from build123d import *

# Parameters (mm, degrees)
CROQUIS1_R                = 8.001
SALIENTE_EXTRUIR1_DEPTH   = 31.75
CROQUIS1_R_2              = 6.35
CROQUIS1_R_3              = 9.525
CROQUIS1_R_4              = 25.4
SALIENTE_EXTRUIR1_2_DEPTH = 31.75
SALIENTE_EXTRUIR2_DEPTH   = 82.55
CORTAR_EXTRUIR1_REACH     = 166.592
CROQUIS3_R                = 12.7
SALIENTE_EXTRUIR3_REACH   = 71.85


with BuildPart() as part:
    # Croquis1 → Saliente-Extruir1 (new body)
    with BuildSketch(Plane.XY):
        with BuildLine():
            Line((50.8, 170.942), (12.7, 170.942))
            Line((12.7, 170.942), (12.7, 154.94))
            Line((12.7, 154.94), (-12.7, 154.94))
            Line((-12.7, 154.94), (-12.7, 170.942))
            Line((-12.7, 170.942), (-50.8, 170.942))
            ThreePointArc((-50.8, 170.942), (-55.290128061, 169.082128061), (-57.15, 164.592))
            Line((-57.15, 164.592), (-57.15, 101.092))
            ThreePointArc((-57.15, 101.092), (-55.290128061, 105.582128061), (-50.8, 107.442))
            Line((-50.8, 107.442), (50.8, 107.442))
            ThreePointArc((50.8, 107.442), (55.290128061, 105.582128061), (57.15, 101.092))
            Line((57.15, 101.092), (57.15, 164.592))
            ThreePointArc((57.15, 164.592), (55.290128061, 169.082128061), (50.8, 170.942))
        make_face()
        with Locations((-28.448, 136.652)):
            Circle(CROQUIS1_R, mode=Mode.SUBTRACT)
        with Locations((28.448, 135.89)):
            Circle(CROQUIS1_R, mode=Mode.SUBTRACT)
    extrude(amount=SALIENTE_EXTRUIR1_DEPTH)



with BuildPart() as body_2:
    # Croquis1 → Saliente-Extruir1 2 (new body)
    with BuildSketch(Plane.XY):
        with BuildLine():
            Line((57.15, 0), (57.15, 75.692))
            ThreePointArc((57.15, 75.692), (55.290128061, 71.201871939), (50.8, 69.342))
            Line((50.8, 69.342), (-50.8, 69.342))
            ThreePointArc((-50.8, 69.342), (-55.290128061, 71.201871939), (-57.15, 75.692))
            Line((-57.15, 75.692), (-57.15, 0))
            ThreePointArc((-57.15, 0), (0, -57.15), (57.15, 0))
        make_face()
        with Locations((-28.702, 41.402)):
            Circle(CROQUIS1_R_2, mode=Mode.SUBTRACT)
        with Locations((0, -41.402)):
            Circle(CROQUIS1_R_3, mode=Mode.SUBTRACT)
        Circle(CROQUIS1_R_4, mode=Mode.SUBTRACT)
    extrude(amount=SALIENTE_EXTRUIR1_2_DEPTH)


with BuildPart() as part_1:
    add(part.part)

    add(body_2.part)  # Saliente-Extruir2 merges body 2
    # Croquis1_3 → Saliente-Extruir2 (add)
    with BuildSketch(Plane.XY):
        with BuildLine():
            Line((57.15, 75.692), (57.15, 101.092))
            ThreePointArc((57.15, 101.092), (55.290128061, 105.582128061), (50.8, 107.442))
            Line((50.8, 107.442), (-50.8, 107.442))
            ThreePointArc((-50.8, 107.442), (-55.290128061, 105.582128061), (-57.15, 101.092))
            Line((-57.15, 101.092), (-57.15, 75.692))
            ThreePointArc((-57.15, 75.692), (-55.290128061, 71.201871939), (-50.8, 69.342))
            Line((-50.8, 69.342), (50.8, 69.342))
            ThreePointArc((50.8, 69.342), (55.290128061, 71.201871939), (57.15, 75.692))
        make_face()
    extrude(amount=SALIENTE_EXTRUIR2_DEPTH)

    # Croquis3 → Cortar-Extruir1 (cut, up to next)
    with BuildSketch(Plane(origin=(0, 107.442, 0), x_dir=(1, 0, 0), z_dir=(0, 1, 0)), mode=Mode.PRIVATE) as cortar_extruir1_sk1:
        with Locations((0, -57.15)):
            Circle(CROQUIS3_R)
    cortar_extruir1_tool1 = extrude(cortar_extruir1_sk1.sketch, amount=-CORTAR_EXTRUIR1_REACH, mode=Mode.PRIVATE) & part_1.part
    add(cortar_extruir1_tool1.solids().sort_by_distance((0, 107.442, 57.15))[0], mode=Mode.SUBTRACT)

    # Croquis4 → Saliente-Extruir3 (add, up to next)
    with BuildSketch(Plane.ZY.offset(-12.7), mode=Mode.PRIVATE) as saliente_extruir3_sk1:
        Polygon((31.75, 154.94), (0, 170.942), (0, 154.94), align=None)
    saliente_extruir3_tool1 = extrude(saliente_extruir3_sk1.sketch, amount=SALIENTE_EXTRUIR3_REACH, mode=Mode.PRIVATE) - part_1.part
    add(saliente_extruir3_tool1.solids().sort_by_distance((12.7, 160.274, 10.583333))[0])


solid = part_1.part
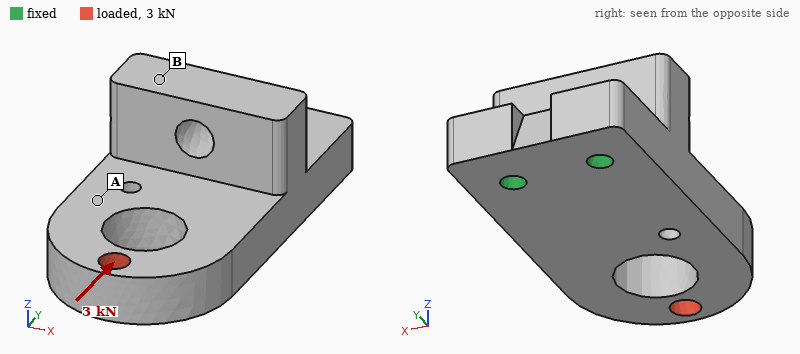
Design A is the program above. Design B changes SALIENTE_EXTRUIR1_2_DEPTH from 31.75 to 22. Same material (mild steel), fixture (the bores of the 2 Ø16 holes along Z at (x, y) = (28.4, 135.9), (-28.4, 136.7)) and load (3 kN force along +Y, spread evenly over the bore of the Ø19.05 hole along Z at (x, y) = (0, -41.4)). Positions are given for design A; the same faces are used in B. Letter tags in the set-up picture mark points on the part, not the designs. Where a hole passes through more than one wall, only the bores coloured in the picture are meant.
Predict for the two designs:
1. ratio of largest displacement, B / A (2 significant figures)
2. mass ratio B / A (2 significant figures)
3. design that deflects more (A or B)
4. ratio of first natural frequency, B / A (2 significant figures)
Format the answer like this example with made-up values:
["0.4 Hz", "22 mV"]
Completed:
["1.7", "0.88", "B", "0.99"]
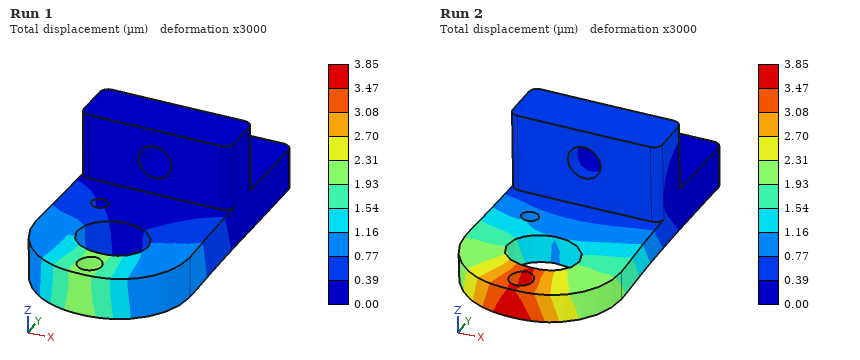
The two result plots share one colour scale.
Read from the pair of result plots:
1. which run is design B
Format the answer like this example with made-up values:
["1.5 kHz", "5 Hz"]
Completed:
["Run 2"]
